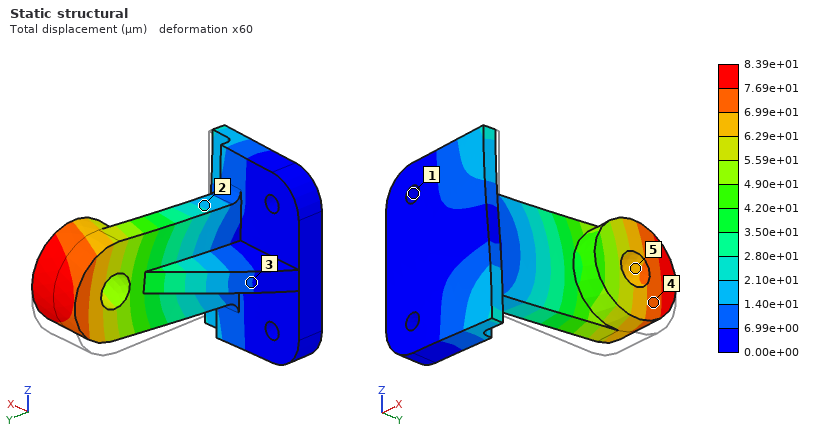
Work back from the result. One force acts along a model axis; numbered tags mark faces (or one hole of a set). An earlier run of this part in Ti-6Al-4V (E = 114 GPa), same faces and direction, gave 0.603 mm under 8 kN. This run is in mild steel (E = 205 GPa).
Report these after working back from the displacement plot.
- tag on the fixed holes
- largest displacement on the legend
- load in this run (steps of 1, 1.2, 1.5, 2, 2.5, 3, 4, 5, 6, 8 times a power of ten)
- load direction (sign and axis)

1
8.39e+01 µm
2 kN
+Z
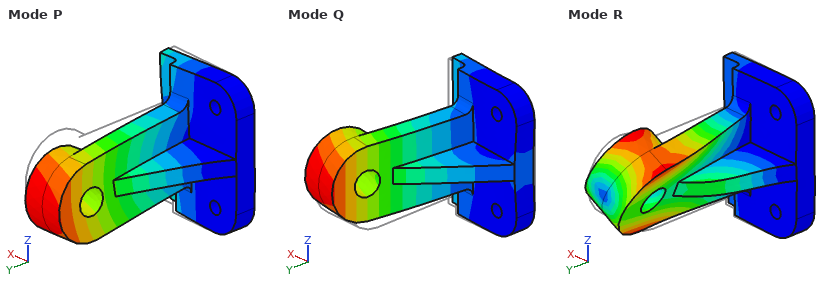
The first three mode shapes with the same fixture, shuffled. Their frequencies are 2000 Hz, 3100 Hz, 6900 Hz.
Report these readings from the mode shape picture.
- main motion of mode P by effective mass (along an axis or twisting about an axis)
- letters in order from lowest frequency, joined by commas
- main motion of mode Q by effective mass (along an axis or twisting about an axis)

along Z
Q, P, R
along X
